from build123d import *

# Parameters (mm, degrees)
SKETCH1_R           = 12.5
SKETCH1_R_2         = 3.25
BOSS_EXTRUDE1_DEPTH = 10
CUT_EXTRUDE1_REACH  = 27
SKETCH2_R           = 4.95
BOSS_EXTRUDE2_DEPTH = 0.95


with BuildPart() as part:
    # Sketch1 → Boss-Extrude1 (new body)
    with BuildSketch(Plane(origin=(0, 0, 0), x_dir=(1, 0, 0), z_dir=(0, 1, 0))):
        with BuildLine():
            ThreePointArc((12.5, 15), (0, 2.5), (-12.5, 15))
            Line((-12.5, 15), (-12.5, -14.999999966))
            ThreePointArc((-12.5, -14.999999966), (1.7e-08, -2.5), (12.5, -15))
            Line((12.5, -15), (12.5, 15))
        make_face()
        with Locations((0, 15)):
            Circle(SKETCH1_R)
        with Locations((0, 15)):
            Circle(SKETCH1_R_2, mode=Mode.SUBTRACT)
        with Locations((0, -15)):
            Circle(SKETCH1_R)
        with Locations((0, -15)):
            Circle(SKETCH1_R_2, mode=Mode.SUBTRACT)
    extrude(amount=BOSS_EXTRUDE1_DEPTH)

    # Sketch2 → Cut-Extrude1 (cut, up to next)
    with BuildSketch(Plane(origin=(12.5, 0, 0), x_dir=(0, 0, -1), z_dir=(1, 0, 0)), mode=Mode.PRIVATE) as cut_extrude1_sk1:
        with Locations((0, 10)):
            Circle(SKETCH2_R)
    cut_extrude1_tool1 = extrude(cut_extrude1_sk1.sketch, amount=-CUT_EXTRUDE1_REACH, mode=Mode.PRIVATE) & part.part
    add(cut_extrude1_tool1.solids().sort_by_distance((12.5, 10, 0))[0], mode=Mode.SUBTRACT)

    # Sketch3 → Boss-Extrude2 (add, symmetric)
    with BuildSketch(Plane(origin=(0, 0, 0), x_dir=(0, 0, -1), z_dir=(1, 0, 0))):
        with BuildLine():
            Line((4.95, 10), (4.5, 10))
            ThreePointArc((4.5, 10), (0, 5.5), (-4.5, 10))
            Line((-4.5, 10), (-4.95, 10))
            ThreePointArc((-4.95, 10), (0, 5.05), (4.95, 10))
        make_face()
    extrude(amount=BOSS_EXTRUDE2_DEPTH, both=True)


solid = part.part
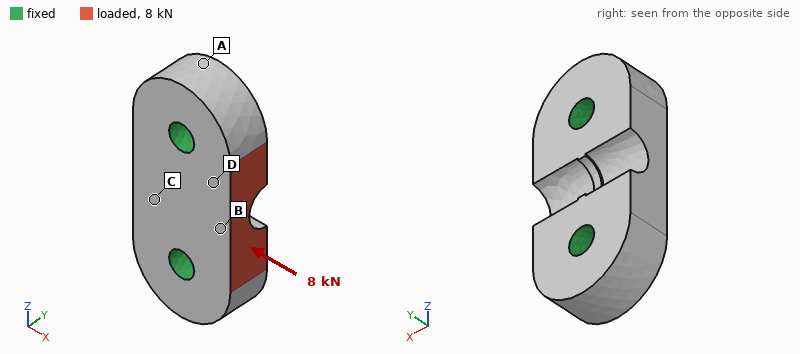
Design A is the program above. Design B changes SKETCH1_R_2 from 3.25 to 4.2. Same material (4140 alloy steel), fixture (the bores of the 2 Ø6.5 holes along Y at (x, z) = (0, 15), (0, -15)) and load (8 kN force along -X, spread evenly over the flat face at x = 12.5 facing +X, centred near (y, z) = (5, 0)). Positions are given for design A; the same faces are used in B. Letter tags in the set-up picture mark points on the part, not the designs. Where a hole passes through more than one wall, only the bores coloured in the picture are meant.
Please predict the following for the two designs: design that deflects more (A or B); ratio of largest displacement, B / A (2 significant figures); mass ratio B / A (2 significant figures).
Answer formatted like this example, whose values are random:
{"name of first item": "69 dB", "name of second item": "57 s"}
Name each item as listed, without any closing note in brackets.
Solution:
{"design that deflects more": "A", "ratio of largest displacement, B / A": "0.86", "mass ratio B / A": "0.96"}
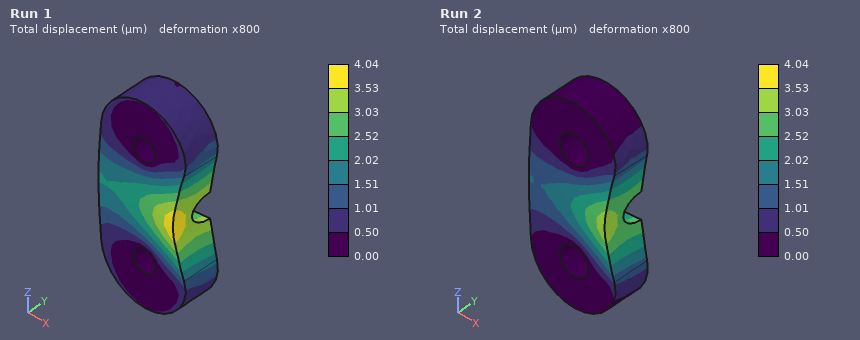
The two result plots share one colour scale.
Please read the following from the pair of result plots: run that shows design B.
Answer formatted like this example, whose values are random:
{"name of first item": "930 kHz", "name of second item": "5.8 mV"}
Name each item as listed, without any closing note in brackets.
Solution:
{"run that shows design B": "Run 2"}
